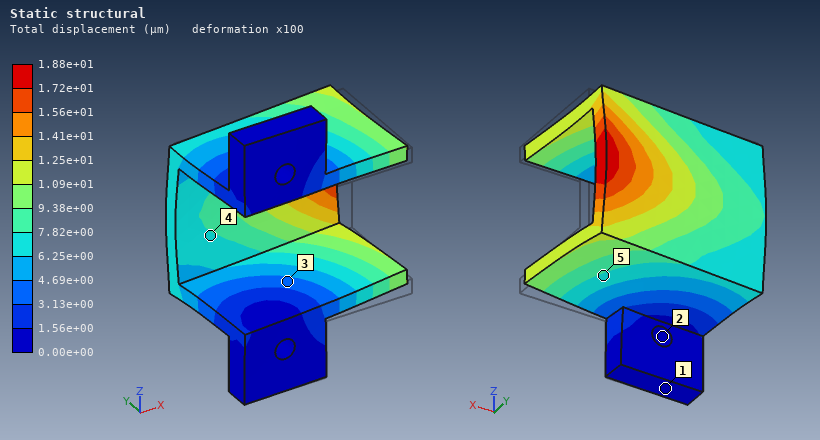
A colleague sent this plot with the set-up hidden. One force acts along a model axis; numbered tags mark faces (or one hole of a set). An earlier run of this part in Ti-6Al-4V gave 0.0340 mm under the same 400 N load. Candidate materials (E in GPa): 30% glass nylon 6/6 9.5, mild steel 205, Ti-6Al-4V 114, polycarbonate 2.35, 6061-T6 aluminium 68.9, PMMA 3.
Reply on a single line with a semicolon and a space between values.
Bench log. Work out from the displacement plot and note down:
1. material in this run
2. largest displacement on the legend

mild steel; 1.88e+01 µm
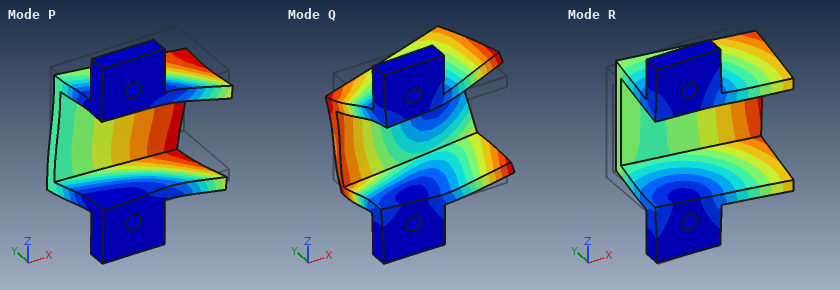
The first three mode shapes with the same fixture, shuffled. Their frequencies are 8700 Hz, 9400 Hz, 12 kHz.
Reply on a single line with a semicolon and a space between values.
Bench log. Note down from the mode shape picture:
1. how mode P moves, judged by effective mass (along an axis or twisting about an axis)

along Z
